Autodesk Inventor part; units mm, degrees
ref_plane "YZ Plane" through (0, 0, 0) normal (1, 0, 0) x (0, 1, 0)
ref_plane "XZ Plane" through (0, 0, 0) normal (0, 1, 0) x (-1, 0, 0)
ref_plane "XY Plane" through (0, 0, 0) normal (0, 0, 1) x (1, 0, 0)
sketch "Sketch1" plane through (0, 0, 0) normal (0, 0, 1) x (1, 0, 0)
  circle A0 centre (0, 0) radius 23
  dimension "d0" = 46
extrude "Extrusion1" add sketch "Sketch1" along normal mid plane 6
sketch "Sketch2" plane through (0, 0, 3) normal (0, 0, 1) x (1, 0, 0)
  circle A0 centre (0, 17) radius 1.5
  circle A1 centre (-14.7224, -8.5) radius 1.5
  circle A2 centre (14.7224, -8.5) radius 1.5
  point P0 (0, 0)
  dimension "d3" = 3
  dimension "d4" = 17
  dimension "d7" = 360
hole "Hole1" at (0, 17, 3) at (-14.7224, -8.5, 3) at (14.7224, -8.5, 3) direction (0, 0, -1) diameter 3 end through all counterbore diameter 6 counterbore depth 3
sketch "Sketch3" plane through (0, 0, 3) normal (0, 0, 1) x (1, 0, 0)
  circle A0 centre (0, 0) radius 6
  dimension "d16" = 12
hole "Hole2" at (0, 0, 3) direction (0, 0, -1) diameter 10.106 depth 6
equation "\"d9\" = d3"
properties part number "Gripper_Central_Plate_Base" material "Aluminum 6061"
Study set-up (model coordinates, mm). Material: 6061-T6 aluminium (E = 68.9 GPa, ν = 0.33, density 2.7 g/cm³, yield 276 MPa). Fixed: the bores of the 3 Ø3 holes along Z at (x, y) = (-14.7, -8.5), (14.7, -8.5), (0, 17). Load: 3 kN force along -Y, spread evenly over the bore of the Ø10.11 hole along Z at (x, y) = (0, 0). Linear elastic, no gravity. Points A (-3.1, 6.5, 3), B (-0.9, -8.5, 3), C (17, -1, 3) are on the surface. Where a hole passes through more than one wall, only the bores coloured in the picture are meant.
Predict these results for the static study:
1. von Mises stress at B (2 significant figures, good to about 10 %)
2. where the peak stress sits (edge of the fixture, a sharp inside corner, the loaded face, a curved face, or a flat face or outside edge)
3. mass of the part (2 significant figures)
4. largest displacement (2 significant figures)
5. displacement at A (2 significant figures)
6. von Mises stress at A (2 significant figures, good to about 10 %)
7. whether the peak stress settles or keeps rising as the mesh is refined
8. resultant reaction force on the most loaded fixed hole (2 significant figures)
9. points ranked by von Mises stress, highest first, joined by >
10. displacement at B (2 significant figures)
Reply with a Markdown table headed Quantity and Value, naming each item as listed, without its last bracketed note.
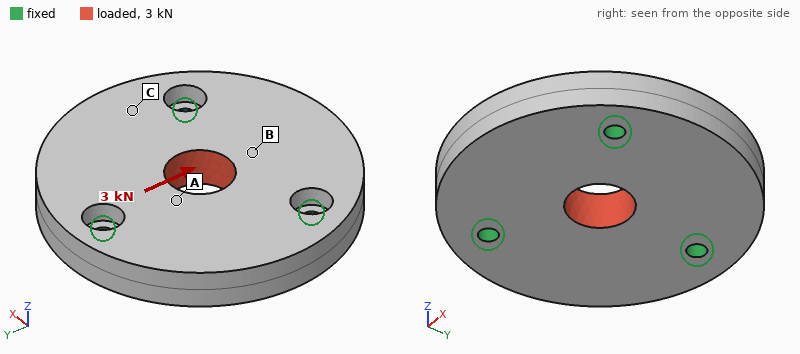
| Quantity | Value |
|---|---|
| von Mises stress at B | 11 MPa |
| where the peak stress sits | edge of the fixture |
| mass of the part | 25 g |
| largest displacement | 8.0 µm |
| displacement at A | 4.0 µm |
| von Mises stress at A | 22 MPa |
| whether the peak stress settles or keeps rising as the mesh is refined | keeps rising |
| resultant reaction force on the most loaded fixed hole | 1.1 kN |
| points ranked by von Mises stress, highest first, joined by > | A > B > C |
| displacement at B | 6.3 µm |
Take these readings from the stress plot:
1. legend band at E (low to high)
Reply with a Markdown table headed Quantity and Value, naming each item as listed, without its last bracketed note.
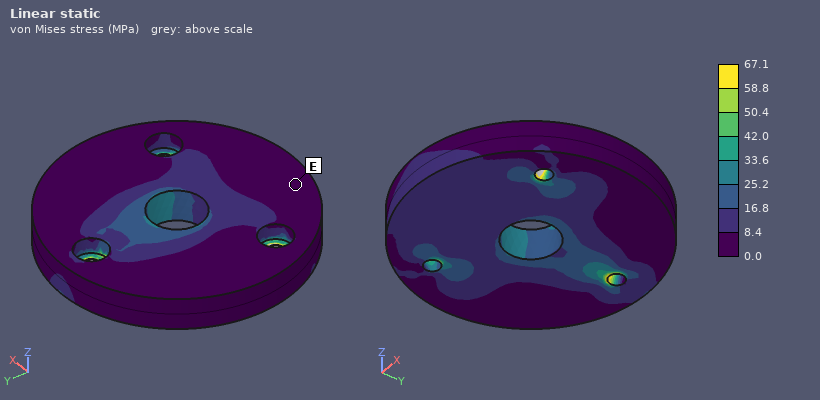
| Quantity | Value |
|---|---|
| legend band at E | 0.0 to 8.4 MPa |
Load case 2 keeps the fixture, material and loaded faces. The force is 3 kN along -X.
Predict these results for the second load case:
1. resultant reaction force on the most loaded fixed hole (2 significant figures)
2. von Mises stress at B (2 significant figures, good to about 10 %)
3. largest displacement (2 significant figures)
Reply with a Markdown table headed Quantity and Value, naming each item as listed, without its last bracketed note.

| Quantity | Value |
|---|---|
| resultant reaction force on the most loaded fixed hole | 1.0 kN |
| von Mises stress at B | 13 MPa |
| largest displacement | 6.9 µm |
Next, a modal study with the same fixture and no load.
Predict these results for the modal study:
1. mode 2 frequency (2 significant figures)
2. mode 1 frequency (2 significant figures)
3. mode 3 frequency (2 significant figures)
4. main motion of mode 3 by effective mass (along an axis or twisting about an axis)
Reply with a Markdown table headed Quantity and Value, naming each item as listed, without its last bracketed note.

| Quantity | Value |
|---|---|
| mode 2 frequency | 12 kHz |
| mode 1 frequency | 12 kHz |
| mode 3 frequency | 17 kHz |
| main motion of mode 3 by effective mass | along Z |
